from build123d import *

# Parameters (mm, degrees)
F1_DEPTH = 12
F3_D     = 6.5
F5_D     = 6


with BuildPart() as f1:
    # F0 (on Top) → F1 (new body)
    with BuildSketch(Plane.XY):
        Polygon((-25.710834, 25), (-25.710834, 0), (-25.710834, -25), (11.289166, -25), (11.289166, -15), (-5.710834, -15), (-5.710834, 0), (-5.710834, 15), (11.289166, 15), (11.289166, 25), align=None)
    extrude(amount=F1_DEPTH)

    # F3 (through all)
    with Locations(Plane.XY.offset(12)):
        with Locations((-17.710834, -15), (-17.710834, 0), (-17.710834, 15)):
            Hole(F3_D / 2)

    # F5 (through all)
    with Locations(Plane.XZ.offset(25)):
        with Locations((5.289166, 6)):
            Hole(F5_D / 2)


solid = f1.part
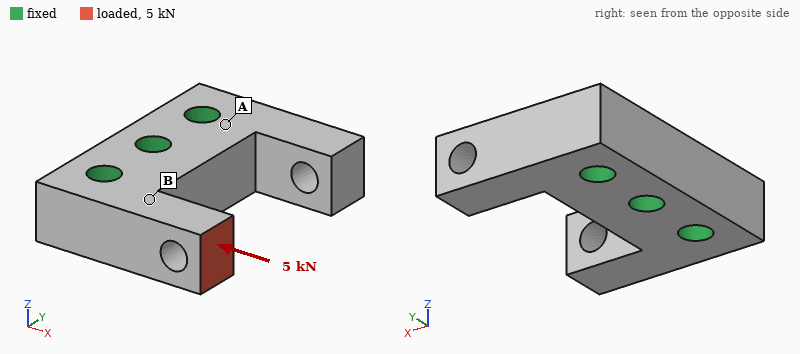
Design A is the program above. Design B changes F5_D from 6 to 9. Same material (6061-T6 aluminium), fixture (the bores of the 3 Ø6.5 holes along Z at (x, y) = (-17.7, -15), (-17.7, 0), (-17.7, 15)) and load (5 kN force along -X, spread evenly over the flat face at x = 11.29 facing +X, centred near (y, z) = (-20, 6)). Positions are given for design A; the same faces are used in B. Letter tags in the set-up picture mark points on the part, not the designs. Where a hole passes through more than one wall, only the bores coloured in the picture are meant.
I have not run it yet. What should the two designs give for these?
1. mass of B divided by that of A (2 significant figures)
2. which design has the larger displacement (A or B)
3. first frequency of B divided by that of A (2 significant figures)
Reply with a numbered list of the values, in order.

1. 0.95
2. B
3. 1.0
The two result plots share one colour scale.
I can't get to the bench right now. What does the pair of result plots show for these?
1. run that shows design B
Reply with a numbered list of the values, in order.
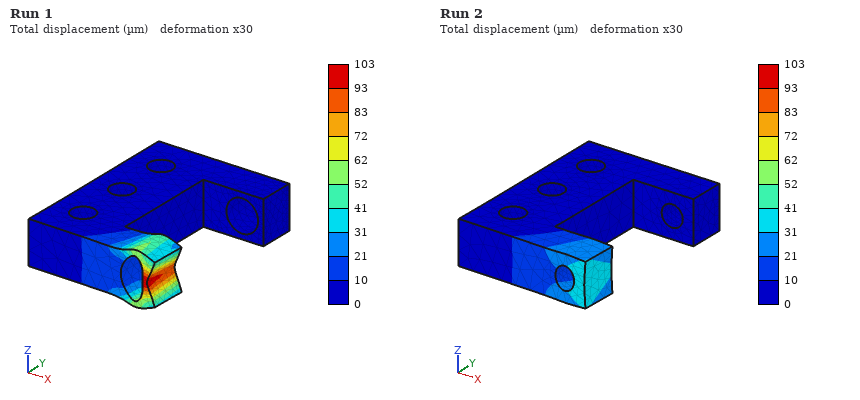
1. Run 1
